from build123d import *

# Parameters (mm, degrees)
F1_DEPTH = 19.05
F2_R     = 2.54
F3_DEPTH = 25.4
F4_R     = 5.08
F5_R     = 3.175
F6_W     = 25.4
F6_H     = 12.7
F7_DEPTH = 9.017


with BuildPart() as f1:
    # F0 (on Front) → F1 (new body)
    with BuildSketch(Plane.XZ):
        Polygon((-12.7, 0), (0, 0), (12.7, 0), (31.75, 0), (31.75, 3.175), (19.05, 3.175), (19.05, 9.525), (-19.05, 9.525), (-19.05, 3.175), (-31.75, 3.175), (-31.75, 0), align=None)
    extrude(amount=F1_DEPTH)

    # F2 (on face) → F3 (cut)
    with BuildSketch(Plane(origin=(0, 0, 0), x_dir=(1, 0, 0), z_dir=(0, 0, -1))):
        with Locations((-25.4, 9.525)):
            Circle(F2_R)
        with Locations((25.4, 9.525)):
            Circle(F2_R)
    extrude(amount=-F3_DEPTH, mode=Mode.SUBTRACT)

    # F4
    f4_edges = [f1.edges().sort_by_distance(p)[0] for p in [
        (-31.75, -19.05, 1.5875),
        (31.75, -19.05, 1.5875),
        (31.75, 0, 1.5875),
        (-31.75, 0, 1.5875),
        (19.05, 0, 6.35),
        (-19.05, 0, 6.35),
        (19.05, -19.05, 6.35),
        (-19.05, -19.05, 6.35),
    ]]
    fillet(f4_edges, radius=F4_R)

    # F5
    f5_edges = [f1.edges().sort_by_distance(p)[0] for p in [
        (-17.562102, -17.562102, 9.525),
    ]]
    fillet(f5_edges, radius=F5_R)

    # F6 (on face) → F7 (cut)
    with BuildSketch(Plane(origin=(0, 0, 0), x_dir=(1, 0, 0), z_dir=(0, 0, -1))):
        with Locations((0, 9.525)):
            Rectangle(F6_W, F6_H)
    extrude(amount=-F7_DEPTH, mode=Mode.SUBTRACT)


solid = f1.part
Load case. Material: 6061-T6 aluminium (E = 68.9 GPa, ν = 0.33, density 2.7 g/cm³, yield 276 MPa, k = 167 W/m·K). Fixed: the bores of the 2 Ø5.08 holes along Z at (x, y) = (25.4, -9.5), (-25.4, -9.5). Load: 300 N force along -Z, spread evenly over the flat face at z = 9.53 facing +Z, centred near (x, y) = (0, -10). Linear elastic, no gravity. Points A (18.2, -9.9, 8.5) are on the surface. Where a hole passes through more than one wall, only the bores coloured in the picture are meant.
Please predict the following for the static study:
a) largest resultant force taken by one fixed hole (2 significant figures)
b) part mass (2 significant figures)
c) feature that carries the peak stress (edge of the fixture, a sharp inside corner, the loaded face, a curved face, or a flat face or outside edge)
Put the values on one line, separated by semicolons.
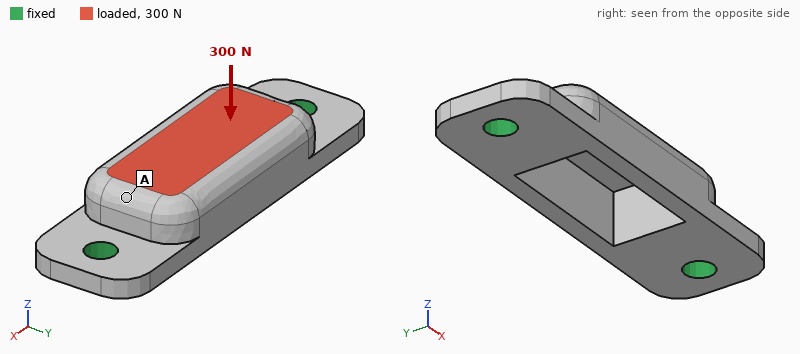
230 N; 13 g; the loaded face
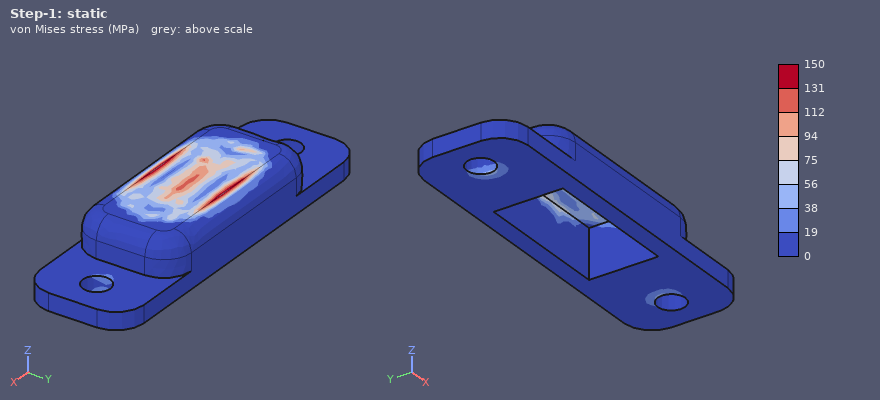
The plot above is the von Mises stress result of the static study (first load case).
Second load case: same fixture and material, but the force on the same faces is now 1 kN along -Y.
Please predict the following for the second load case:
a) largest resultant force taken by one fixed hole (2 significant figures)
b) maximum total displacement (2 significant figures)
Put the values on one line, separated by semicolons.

500 N; 53 µm
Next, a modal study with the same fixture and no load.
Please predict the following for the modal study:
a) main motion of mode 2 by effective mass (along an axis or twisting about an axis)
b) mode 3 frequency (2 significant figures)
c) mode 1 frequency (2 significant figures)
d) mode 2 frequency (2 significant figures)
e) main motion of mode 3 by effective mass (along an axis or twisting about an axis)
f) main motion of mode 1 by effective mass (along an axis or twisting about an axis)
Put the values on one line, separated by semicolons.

along Z; 18 kHz; 9100 Hz; 12 kHz; along Y; along Y
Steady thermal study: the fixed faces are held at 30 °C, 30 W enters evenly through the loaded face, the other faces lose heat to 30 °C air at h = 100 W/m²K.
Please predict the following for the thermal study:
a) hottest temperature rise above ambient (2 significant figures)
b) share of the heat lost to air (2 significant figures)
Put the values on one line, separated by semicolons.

38 K; 15 %
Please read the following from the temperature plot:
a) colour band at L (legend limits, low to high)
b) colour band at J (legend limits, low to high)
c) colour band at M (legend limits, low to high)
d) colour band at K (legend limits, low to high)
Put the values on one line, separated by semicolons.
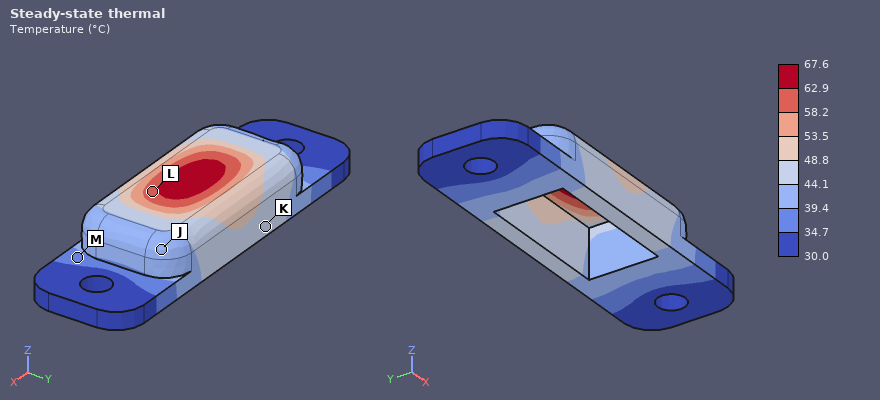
58.2 to 62.9 °C; 39.4 to 44.1 °C; 34.7 to 39.4 °C; 44.1 to 48.8 °C
